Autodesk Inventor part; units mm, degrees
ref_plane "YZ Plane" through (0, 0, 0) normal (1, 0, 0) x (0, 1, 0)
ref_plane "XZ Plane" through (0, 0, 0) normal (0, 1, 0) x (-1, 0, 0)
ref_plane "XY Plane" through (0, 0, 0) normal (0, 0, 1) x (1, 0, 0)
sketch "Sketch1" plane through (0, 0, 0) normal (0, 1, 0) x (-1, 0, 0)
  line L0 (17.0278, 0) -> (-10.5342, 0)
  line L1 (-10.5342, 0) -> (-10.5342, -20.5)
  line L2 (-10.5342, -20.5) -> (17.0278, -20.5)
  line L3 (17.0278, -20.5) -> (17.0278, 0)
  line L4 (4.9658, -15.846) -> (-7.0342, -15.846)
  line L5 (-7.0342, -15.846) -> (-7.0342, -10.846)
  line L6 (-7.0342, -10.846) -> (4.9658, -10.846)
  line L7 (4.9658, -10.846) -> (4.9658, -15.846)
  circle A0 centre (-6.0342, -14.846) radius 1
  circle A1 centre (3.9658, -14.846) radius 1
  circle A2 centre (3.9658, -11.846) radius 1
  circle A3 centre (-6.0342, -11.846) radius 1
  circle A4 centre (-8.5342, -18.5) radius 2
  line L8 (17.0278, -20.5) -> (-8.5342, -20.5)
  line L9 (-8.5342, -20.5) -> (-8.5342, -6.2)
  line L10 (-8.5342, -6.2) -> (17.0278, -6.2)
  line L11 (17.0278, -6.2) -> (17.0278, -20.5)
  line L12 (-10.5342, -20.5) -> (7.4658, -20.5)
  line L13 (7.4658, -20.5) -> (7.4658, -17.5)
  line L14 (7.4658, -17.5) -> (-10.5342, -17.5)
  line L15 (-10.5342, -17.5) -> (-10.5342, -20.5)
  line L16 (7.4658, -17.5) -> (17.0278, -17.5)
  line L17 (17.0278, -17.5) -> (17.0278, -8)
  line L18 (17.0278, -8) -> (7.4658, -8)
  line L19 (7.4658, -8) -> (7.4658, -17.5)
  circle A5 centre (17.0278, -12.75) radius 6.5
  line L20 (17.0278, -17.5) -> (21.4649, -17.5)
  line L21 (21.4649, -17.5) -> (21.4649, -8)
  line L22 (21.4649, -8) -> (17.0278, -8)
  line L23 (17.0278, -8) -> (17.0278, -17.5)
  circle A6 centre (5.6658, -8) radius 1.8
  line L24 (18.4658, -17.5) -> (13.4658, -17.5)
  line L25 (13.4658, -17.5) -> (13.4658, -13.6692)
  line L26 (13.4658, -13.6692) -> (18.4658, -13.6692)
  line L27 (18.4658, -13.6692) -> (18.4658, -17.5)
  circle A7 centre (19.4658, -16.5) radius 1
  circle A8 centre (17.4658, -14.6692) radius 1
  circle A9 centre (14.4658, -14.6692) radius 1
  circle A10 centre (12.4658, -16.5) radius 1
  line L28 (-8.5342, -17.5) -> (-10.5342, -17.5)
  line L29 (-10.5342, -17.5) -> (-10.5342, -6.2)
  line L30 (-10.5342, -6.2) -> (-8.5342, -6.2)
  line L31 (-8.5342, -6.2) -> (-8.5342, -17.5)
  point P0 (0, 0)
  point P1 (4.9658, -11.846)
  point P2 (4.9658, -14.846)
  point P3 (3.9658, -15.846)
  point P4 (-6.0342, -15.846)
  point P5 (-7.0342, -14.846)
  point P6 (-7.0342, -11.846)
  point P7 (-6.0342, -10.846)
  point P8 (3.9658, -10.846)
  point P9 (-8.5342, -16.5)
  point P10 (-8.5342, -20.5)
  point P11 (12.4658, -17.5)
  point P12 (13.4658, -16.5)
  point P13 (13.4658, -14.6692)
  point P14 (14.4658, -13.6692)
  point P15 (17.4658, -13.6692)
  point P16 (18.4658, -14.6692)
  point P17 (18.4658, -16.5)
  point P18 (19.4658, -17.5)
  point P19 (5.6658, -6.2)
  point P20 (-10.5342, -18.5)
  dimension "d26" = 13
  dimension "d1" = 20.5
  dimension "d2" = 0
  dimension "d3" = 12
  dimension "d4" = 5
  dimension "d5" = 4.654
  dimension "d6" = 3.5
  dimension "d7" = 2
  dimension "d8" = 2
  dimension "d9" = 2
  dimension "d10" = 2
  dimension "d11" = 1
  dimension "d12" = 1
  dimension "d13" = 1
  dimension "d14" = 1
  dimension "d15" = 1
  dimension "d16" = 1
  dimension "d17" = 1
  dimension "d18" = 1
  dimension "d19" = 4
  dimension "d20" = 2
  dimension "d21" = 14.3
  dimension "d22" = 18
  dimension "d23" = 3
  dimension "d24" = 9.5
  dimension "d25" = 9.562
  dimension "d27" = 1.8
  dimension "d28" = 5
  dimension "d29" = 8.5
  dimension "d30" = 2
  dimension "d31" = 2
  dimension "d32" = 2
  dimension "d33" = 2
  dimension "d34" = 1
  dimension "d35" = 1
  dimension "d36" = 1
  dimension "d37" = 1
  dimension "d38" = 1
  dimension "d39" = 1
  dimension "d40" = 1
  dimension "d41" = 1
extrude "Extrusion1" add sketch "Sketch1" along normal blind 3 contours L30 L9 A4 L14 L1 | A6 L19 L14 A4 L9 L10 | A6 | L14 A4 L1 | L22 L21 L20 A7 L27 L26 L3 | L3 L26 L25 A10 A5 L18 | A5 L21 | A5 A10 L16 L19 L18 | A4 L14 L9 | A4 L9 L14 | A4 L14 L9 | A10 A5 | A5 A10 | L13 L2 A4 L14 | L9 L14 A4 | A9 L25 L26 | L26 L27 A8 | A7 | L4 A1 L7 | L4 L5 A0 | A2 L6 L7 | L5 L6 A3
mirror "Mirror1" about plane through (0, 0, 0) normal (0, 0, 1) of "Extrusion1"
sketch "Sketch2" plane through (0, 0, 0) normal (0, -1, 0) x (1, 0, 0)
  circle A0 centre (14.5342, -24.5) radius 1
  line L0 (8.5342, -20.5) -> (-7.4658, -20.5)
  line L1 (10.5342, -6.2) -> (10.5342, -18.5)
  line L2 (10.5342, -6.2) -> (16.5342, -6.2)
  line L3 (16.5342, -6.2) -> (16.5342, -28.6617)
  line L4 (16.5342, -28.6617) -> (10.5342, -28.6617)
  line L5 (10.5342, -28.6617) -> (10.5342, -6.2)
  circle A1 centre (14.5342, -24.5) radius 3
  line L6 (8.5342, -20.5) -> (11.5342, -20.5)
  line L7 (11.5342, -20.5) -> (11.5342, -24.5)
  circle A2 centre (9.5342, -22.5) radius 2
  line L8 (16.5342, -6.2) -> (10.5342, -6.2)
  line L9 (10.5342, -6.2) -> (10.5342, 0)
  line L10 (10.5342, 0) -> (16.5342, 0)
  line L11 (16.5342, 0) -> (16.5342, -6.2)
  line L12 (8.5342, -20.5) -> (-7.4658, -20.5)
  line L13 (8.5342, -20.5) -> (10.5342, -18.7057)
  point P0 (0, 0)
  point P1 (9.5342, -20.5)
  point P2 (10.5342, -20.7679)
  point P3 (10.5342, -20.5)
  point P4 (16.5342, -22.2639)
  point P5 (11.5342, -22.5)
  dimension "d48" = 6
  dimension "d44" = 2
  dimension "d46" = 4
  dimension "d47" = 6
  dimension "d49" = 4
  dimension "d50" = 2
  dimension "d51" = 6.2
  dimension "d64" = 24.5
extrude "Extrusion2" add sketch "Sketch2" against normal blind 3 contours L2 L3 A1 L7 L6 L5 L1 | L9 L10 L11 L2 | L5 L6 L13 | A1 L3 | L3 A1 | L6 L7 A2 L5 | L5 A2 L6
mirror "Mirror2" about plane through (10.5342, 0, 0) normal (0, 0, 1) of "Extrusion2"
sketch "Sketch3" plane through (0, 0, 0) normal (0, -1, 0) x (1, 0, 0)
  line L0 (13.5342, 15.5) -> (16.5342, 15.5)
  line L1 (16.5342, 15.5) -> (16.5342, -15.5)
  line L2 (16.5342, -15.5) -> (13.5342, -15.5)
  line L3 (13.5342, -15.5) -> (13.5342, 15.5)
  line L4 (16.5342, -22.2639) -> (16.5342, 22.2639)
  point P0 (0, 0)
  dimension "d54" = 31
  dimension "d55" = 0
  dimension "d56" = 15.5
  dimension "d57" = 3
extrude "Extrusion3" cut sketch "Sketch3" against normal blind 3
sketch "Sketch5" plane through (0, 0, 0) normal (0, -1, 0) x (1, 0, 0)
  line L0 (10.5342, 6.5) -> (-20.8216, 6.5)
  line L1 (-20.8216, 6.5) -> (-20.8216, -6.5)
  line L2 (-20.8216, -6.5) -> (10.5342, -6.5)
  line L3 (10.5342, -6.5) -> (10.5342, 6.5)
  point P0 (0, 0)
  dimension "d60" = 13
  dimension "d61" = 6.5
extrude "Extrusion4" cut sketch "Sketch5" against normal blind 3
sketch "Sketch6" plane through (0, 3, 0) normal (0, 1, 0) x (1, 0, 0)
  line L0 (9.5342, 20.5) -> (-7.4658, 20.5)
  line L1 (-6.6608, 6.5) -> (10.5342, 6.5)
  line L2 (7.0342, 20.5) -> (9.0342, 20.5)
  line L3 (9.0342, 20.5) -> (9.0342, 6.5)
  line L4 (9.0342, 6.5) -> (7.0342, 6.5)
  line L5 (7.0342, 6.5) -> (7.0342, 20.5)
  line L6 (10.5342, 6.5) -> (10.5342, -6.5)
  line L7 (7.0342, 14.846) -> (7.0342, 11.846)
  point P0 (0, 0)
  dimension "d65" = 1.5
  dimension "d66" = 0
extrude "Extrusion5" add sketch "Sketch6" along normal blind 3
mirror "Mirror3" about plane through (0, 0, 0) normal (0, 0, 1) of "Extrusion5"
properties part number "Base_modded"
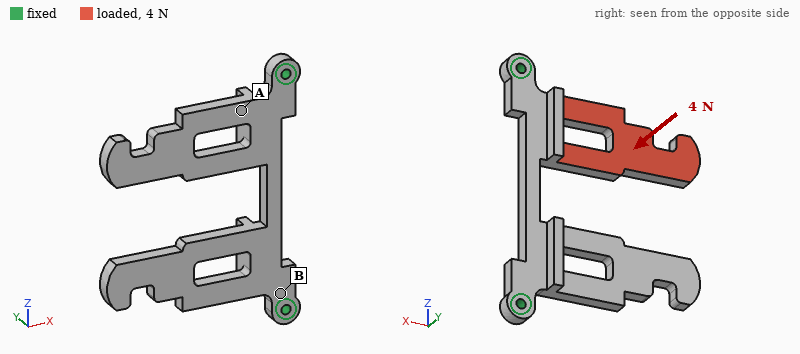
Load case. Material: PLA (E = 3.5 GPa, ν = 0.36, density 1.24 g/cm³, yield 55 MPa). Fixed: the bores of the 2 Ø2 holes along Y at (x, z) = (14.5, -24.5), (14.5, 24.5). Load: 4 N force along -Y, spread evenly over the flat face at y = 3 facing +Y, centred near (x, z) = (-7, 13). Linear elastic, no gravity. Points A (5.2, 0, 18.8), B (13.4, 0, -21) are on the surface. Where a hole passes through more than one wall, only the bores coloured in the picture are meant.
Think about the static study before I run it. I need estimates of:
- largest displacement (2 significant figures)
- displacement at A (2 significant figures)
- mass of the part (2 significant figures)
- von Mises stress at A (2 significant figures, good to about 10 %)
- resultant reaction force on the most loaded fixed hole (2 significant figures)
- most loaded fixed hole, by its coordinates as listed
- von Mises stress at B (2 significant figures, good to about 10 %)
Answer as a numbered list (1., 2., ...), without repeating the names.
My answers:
1. 0.76 mm
2. 0.12 mm
3. 3.4 g
4. 3.9 MPa
5. 3.3 N
6. (14.5, 24.5)
7. 2.0 MPa
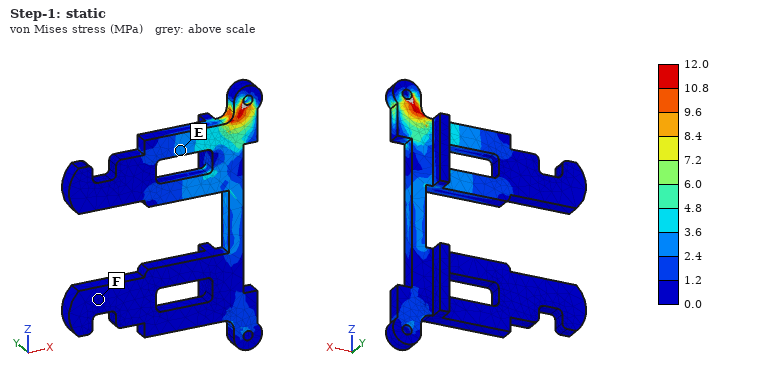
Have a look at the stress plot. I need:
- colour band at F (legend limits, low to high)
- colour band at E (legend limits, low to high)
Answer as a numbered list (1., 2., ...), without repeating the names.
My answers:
1. 0.0 to 1.2 MPa
2. 2.4 to 3.6 MPa
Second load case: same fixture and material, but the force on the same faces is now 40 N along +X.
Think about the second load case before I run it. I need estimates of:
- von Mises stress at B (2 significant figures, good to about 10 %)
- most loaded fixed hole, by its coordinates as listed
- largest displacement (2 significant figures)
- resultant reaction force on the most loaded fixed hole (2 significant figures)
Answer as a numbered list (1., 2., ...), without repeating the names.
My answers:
1. 2.0 MPa
2. (14.5, 24.5)
3. 0.79 mm
4. 41 N
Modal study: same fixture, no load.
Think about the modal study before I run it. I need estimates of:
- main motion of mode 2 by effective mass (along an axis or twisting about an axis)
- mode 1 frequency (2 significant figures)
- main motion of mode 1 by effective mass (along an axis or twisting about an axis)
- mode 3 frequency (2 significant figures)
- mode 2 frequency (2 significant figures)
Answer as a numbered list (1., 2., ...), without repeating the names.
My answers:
1. twisting about X
2. 420 Hz
3. along Y
4. 860 Hz
5. 490 Hz
